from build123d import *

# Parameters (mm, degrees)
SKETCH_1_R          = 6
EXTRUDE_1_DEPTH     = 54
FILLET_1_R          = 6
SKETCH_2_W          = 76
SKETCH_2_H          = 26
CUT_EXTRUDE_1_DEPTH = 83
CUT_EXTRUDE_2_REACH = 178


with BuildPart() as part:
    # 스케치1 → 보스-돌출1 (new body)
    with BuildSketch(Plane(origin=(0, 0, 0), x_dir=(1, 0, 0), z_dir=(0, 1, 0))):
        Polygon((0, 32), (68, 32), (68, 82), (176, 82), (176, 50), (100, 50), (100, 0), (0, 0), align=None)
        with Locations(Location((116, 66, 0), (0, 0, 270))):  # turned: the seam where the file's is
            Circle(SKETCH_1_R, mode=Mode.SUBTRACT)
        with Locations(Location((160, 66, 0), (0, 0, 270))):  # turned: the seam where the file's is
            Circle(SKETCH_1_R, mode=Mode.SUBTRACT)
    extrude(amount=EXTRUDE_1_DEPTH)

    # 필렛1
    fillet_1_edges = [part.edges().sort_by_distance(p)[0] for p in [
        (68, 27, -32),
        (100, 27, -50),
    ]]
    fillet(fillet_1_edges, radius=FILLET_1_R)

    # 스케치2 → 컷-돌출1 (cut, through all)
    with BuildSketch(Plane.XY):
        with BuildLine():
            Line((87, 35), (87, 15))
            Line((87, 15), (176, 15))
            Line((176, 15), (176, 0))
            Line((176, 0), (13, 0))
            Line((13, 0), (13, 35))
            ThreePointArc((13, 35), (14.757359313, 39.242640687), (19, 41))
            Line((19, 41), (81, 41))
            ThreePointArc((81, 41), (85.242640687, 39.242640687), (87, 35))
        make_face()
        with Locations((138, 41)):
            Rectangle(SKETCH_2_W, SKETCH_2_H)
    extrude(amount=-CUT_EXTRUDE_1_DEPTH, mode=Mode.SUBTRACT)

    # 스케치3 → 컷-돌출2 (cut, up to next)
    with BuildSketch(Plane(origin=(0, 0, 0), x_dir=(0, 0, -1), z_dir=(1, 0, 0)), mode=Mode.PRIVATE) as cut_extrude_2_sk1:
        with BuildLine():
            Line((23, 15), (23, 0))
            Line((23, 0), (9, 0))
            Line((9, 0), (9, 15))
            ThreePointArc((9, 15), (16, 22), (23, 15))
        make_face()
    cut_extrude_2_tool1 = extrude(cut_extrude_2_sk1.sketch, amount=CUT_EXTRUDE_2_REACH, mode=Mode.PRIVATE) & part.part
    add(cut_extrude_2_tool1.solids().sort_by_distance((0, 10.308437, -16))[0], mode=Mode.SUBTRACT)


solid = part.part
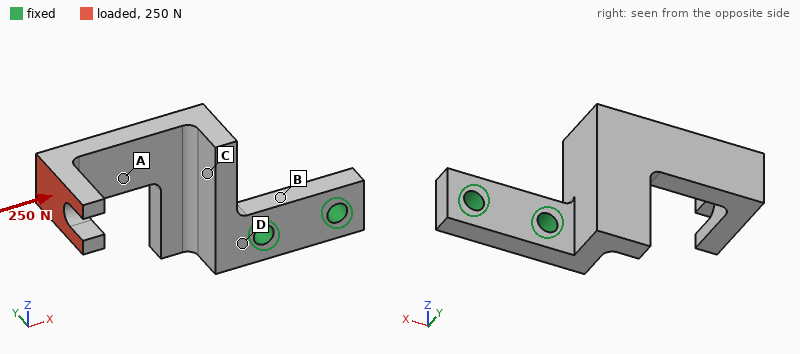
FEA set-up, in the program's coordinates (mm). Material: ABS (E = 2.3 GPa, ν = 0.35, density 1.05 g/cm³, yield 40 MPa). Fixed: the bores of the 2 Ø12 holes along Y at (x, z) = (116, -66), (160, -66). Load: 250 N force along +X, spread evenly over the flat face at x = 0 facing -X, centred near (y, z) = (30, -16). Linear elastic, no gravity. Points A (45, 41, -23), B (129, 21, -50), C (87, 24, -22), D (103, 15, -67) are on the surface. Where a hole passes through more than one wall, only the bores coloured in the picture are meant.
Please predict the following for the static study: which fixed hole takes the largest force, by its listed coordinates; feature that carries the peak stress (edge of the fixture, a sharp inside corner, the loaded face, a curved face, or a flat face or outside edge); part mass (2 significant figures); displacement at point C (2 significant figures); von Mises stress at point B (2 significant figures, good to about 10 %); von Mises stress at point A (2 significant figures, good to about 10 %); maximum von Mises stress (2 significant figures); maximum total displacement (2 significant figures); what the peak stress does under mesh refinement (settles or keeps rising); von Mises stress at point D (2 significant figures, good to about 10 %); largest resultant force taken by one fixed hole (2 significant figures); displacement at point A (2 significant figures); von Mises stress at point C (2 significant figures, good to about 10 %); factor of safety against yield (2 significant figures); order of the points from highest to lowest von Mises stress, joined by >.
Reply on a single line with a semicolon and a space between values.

(116, -66); a curved face; 140 g; 0.44 mm; 1.7 MPa; 5.4 MPa; 21 MPa; 2.2 mm; settles; 4.4 MPa; 260 N; 0.78 mm; 0.82 MPa; 1.9; A > D > B > C
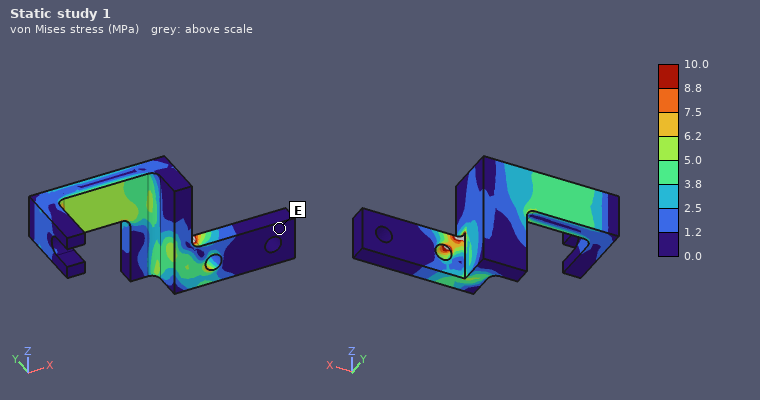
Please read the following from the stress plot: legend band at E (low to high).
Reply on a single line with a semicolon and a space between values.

0.0 to 1.2 MPa
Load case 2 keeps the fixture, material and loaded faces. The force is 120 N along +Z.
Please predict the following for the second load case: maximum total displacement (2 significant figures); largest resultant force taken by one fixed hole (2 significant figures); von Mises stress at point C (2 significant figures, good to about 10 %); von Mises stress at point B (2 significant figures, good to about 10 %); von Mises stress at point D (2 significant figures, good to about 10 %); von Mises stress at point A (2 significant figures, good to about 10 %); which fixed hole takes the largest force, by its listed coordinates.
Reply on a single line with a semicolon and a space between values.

2.4 mm; 240 N; 1.6 MPa; 1.7 MPa; 3.7 MPa; 3.2 MPa; (116, -66)
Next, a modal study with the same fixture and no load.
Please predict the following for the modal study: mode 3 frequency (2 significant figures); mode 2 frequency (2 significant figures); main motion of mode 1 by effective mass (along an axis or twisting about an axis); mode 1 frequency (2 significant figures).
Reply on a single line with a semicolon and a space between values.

440 Hz; 230 Hz; along Y; 140 Hz
